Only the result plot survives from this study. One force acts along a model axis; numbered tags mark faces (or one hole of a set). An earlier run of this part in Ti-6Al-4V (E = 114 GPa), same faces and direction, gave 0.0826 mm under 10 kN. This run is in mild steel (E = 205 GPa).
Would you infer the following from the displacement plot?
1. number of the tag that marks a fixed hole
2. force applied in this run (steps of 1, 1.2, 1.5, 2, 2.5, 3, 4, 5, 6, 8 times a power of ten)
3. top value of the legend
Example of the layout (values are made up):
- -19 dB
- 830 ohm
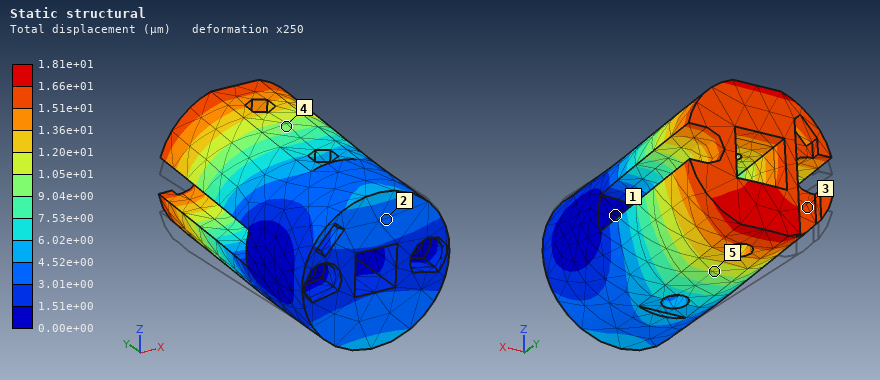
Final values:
- 1
- 4 kN
- 1.81e+01 µm
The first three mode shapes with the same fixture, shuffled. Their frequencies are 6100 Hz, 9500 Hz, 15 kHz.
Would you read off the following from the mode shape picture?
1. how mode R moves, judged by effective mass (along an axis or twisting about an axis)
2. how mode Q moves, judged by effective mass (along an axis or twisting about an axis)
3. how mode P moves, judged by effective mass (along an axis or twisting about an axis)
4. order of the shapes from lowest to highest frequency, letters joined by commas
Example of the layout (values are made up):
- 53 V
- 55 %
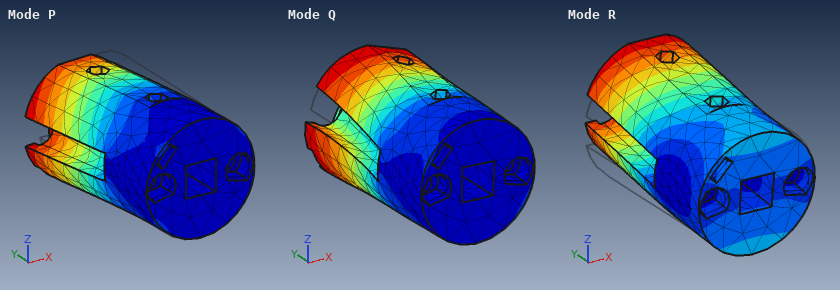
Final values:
- along Z
- twisting about Y
- along X
- R, P, Q
